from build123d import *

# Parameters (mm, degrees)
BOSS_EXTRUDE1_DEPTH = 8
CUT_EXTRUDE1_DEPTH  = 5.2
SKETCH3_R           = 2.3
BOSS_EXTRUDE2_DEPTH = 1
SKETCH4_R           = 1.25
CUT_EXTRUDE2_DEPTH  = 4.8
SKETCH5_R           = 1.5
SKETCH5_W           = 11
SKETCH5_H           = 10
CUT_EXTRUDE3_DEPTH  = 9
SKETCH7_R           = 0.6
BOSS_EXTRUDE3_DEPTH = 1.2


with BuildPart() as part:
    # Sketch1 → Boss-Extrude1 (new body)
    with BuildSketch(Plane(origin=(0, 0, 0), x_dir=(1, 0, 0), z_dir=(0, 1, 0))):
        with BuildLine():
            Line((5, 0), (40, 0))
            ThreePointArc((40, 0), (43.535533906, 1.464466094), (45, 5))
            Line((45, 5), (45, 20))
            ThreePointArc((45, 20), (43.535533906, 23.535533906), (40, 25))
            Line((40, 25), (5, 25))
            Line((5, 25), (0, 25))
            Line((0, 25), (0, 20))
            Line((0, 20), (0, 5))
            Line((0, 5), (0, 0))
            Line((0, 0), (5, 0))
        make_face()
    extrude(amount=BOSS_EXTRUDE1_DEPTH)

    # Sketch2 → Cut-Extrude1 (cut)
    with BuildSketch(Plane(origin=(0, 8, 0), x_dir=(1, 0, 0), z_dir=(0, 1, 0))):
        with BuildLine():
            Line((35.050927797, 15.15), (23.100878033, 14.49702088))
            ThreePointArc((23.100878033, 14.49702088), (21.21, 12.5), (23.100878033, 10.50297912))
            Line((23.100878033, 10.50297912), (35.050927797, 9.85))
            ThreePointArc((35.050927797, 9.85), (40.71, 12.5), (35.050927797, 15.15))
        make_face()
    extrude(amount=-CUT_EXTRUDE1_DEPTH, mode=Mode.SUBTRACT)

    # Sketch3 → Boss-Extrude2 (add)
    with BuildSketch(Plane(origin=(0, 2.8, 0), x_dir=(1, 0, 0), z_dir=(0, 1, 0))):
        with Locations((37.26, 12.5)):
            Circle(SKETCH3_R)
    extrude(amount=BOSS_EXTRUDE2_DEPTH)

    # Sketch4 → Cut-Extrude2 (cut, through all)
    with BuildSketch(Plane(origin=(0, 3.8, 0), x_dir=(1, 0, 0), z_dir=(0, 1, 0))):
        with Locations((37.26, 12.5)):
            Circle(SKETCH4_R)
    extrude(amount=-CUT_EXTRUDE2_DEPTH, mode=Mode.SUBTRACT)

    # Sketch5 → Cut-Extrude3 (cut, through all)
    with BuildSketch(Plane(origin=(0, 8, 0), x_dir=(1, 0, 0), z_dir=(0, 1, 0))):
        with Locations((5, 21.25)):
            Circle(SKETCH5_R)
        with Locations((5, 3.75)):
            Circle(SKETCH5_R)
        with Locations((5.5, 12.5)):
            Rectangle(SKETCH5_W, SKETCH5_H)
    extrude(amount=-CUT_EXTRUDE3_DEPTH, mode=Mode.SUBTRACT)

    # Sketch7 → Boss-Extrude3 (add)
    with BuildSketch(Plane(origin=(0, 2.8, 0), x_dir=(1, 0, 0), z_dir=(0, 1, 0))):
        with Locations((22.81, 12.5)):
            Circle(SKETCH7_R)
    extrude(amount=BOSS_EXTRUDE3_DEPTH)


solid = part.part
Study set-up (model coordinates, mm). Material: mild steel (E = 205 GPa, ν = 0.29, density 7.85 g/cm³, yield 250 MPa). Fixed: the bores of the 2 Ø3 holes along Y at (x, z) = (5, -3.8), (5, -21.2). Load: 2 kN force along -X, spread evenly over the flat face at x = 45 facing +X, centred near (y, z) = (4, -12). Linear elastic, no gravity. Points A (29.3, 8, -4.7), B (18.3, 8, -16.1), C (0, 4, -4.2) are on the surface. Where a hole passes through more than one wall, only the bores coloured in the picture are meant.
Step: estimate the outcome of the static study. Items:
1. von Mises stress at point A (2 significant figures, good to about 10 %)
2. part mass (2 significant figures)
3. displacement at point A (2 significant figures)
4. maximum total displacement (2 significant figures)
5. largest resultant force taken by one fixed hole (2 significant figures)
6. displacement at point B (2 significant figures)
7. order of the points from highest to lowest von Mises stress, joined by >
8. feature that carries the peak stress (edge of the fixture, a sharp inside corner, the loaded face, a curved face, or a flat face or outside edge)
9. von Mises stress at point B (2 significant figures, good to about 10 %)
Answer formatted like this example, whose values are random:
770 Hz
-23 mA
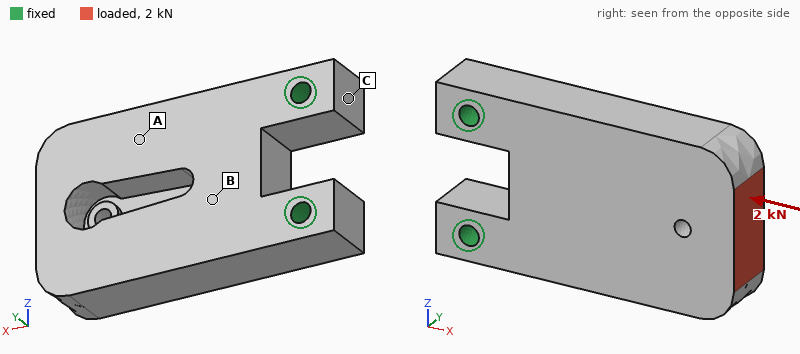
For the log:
14 MPa
58 g
1.7 µm
4.0 µm
1.0 kN
1.0 µm
A > B > C
a curved face
8.6 MPa
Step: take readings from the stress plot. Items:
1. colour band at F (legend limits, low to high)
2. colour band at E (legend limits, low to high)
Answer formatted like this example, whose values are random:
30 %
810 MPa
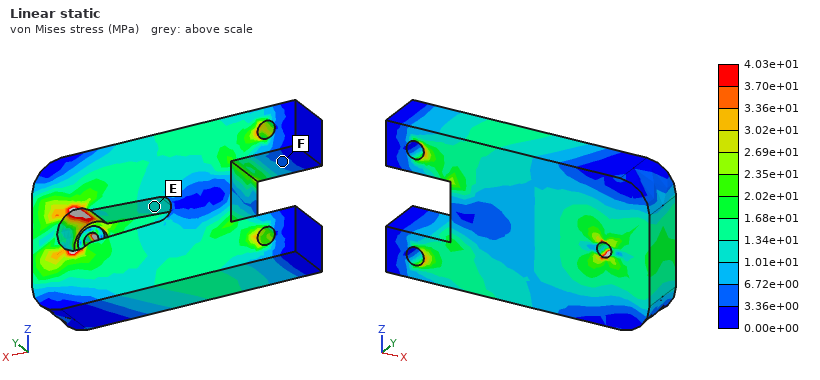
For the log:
3.36e+00 to 6.72e+00 MPa
1.01e+01 to 1.34e+01 MPa
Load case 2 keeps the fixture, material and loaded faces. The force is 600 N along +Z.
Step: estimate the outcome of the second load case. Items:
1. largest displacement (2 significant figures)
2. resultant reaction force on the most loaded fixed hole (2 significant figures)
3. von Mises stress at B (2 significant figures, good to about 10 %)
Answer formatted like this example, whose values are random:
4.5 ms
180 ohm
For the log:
10 µm
1.2 kN
8.9 MPa
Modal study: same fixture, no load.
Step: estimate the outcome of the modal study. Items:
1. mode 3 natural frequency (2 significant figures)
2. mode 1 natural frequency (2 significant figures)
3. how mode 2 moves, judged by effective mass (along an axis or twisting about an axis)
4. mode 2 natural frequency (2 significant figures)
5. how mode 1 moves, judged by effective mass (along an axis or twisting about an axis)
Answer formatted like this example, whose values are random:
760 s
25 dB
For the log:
11 kHz
3600 Hz
along Z
9600 Hz
along Y
